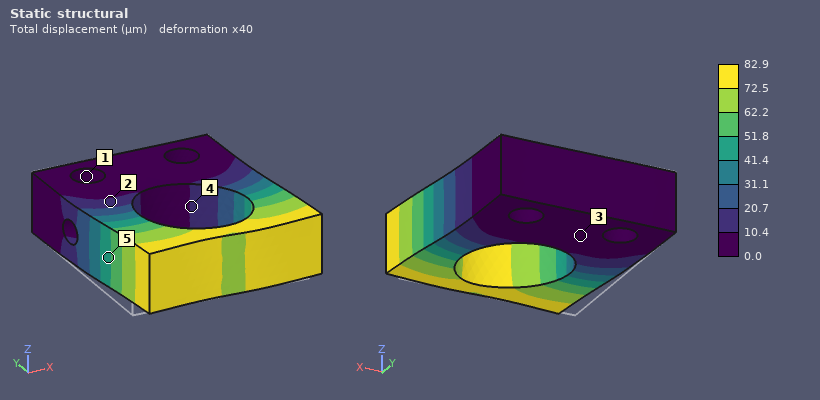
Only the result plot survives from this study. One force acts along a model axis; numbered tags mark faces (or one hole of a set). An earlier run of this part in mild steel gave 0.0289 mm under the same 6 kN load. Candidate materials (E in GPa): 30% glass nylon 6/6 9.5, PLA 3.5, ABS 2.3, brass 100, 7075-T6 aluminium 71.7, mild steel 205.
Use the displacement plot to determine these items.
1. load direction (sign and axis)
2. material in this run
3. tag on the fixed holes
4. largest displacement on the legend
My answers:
+X
7075-T6 aluminium
1
82.9 µm
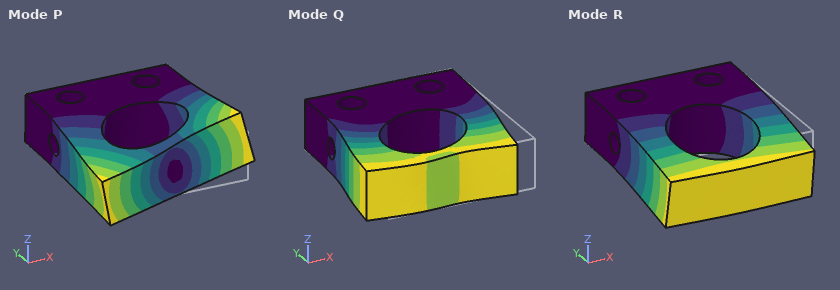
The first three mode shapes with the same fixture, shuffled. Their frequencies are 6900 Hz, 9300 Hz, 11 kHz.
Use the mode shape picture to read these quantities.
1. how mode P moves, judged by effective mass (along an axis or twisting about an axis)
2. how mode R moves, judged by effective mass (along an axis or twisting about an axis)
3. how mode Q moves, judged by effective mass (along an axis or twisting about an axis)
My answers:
twisting about Y
along Z
along X
